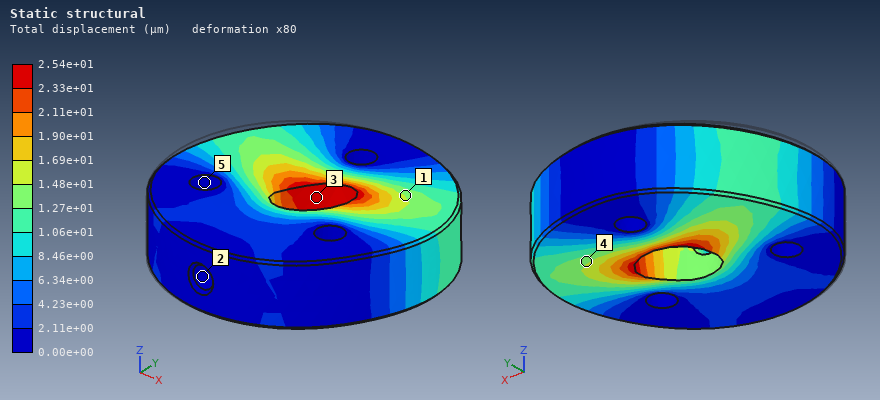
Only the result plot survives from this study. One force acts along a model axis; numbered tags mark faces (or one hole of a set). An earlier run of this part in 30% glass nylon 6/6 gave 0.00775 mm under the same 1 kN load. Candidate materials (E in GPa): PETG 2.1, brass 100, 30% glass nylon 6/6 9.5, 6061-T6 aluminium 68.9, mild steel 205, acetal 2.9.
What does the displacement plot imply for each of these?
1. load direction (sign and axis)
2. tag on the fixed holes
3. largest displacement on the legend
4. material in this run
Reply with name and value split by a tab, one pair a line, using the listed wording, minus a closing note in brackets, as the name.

load direction	+X
tag on the fixed holes	5
largest displacement on the legend	2.54e+01 µm
material in this run	acetal
